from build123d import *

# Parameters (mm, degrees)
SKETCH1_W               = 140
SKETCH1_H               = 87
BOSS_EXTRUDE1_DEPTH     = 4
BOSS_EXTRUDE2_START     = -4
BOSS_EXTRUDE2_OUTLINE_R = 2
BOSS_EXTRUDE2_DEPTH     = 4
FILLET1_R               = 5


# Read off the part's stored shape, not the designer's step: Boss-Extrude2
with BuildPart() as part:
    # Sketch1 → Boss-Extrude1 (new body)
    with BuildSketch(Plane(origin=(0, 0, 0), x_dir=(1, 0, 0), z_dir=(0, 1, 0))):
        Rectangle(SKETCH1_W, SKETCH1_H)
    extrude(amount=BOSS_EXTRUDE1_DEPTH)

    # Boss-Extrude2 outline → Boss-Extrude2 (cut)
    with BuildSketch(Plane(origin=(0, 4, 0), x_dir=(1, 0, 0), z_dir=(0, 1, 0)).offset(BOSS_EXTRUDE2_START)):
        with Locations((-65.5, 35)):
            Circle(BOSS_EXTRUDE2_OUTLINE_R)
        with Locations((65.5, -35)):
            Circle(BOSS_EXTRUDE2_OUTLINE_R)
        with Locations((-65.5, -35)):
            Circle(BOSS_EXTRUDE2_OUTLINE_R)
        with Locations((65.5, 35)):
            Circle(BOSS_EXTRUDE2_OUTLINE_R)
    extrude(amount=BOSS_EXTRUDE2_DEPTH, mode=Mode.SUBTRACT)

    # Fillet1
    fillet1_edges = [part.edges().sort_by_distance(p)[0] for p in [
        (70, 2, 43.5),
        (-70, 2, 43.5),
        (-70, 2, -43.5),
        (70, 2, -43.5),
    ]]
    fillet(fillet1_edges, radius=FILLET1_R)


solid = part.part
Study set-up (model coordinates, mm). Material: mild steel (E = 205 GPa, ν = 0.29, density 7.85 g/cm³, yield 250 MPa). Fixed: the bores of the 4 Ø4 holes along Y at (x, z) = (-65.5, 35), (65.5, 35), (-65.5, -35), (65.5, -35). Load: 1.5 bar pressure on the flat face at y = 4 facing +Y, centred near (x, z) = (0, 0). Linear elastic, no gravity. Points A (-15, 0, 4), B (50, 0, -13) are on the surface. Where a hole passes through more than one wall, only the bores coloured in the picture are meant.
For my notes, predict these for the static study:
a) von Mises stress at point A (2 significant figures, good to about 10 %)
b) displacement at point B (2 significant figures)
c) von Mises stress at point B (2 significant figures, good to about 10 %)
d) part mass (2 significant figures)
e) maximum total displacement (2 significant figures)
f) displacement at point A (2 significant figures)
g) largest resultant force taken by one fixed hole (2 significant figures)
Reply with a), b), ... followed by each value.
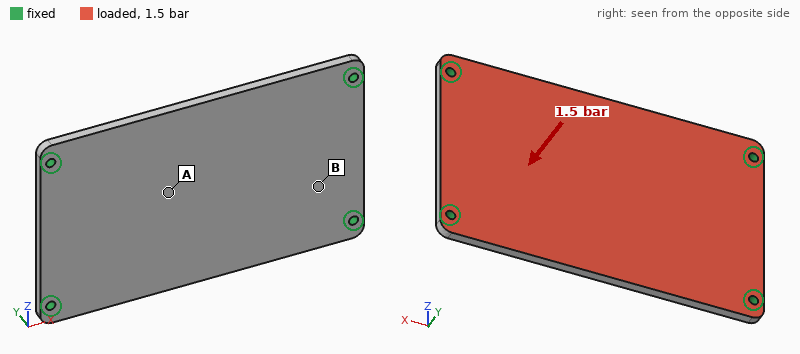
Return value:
a) 38 MPa
b) 0.050 mm
c) 19 MPa
d) 380 g
e) 0.15 mm
f) 0.14 mm
g) 450 N
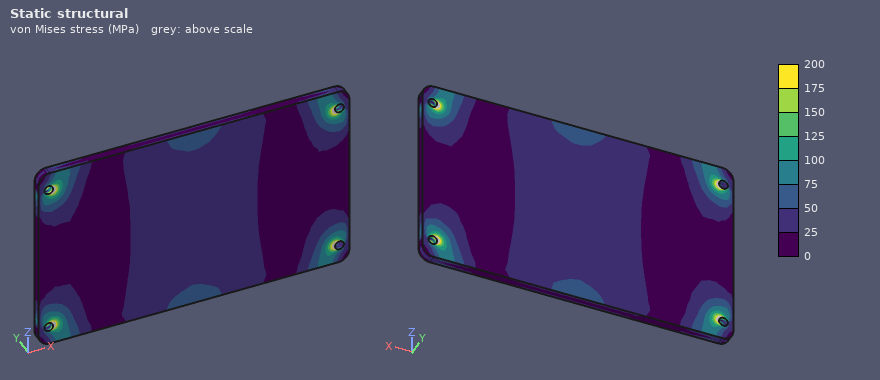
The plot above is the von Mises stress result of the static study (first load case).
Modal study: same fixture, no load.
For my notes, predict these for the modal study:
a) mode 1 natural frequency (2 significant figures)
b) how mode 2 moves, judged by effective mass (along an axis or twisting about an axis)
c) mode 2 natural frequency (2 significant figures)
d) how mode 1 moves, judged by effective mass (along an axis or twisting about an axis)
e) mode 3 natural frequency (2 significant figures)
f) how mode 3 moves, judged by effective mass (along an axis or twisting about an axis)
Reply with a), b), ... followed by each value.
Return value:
a) 1000 Hz
b) twisting about X
c) 1700 Hz
d) along Y
e) 2700 Hz
f) twisting about Z
